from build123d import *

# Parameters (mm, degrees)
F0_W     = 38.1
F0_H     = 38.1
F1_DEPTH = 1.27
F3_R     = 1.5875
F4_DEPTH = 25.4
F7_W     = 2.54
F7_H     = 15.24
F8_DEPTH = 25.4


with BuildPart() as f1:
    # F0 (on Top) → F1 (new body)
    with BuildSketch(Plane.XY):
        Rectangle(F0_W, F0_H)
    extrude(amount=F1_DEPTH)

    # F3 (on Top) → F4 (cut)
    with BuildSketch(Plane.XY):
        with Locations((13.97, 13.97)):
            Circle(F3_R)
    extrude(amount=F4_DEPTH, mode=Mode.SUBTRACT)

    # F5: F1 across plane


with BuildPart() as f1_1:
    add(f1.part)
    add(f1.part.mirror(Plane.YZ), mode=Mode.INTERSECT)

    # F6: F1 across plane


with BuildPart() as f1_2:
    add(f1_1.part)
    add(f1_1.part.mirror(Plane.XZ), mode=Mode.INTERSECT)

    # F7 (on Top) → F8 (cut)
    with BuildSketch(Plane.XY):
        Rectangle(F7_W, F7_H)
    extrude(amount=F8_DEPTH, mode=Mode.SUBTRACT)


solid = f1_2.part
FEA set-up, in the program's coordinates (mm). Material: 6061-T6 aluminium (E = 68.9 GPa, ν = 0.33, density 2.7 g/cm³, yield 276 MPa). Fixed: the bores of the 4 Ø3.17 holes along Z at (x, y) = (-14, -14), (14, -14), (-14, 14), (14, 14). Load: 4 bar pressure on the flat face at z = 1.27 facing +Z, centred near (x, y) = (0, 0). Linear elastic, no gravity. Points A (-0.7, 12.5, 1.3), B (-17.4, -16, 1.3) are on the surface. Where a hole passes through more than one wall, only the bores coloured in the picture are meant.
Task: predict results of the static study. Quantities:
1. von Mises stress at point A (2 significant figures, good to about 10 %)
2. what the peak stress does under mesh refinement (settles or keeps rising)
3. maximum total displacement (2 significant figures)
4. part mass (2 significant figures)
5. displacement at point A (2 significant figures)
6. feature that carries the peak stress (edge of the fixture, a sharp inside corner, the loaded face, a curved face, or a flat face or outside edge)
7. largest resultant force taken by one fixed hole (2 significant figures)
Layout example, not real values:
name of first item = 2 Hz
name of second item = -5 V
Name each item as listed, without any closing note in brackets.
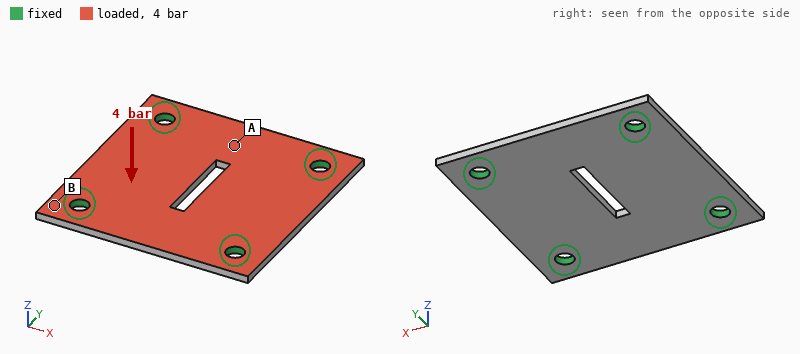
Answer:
von Mises stress at point A = 61 MPa
what the peak stress does under mesh refinement = keeps rising
maximum total displacement = 0.13 mm
part mass = 4.7 g
displacement at point A = 0.066 mm
feature that carries the peak stress = edge of the fixture
largest resultant force taken by one fixed hole = 140 N
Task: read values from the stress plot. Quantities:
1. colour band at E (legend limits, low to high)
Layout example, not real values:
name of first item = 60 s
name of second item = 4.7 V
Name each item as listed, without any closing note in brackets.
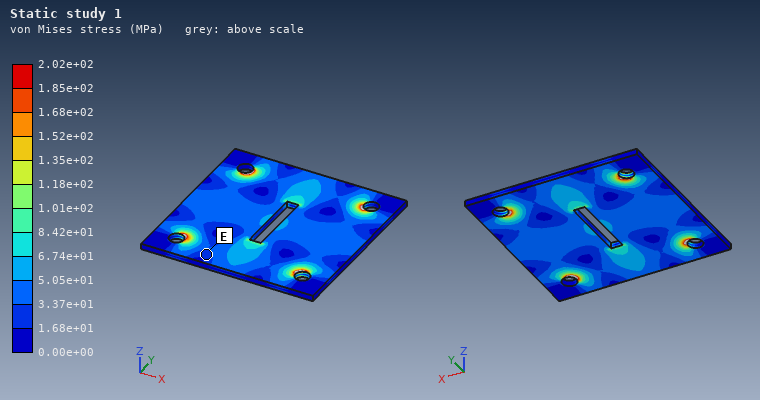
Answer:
colour band at E = 1.68e+01 to 3.37e+01 MPa
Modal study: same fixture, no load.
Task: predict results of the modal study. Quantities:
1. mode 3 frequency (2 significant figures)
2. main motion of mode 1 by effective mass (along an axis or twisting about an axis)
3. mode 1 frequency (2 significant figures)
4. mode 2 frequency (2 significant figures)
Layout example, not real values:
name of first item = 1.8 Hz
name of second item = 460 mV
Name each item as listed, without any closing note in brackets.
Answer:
mode 3 frequency = 10 kHz
main motion of mode 1 by effective mass = along Z
mode 1 frequency = 6300 Hz
mode 2 frequency = 9800 Hz
